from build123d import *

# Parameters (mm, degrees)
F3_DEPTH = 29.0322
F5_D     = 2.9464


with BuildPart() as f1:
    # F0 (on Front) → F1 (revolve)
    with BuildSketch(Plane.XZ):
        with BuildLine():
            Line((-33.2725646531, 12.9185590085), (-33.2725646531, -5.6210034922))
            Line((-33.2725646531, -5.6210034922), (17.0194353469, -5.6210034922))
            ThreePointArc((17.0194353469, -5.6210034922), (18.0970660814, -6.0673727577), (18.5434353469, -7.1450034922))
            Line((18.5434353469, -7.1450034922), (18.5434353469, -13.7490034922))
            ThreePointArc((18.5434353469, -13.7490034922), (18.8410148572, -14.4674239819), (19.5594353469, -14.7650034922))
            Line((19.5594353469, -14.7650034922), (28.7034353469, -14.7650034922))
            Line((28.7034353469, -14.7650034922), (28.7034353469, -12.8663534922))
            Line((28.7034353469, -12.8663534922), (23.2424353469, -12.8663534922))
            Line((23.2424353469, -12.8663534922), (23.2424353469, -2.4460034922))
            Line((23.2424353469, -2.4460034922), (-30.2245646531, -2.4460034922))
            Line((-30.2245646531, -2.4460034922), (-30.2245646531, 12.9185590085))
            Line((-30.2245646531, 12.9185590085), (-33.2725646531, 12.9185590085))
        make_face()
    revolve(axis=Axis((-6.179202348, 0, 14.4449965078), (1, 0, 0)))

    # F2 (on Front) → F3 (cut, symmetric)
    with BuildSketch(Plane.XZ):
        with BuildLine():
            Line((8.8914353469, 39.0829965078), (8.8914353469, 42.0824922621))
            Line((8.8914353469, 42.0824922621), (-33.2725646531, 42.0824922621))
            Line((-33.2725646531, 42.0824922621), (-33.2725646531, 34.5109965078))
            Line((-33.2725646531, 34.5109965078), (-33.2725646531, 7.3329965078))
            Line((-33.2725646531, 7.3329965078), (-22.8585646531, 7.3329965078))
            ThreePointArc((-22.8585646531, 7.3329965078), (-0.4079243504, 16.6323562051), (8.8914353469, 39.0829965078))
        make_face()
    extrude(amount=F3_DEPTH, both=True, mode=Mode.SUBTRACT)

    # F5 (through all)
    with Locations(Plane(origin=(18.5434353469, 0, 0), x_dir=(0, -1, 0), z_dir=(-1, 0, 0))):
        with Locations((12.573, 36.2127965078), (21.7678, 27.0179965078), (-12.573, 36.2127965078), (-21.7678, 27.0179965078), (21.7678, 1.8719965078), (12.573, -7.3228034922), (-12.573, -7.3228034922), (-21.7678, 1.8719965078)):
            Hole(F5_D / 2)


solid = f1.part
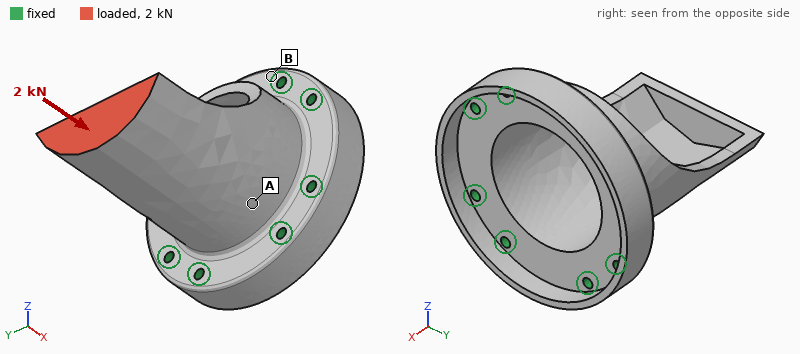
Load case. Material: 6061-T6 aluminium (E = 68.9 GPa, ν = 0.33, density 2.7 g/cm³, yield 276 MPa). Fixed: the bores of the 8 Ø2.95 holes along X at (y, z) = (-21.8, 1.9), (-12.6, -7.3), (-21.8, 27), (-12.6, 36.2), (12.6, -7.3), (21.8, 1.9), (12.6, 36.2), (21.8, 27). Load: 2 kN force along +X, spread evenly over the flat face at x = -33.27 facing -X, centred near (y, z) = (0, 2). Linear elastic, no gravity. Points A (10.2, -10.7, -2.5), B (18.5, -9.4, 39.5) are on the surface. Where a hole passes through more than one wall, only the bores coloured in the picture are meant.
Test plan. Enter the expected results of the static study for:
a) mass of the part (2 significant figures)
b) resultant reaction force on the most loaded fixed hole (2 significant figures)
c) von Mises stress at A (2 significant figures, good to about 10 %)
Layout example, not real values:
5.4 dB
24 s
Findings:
58 g
530 N
12 MPa
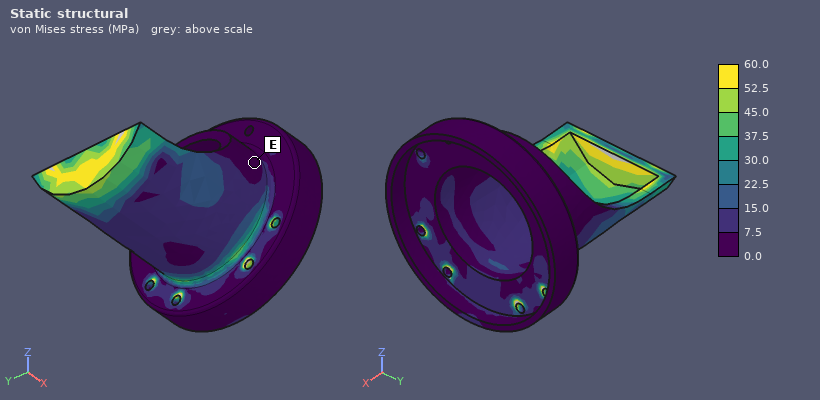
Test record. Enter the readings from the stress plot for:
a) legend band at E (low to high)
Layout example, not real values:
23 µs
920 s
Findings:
0.0 to 7.5 MPa
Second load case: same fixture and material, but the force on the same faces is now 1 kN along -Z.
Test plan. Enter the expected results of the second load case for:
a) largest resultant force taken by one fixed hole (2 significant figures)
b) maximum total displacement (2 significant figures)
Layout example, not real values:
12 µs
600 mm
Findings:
1.0 kN
0.21 mm
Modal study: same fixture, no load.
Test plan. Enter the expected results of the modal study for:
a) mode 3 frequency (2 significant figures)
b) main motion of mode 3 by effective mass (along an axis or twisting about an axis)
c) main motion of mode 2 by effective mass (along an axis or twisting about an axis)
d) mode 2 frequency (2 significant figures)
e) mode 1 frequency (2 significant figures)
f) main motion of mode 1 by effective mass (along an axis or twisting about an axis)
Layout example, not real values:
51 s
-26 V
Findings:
9700 Hz
along Y
along Z
4700 Hz
4100 Hz
along Y
